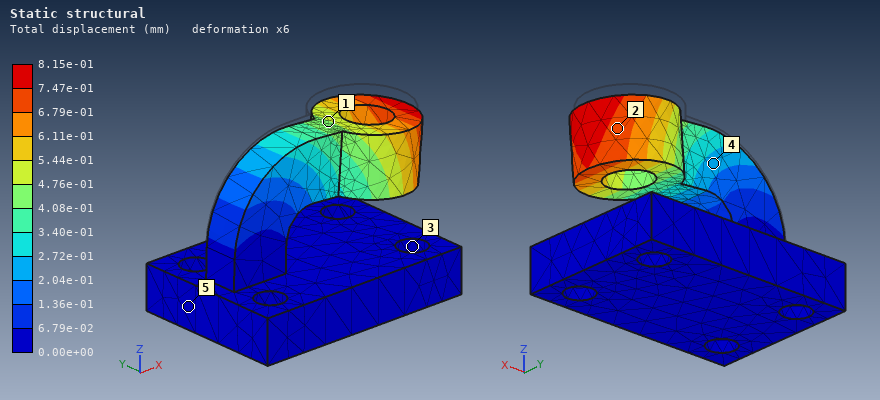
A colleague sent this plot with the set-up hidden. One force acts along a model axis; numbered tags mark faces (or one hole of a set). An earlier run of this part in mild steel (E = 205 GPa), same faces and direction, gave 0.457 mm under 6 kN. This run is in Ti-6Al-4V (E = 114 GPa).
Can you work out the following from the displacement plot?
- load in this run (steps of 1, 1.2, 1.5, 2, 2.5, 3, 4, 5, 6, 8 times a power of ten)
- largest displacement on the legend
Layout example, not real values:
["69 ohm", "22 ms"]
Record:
["6 kN", "8.15e-01 mm"]
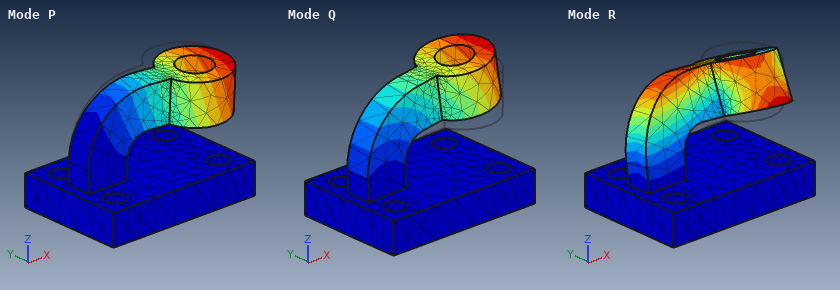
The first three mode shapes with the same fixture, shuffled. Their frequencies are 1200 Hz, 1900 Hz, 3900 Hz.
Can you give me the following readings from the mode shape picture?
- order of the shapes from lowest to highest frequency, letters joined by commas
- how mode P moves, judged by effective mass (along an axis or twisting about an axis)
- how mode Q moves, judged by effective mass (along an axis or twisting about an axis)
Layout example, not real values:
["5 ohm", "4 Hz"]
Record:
["P, Q, R", "along Y", "along Z"]
